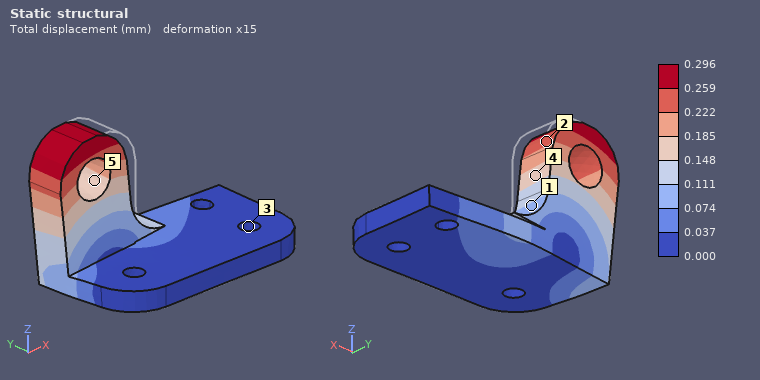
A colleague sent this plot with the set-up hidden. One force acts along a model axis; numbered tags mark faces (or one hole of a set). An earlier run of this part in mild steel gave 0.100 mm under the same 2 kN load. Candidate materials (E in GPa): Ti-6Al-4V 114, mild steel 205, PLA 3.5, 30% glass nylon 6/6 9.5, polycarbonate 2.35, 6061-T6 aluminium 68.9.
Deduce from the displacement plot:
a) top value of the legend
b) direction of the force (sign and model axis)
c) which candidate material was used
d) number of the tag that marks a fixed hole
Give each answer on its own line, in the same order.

0.296 mm
-X
6061-T6 aluminium
3
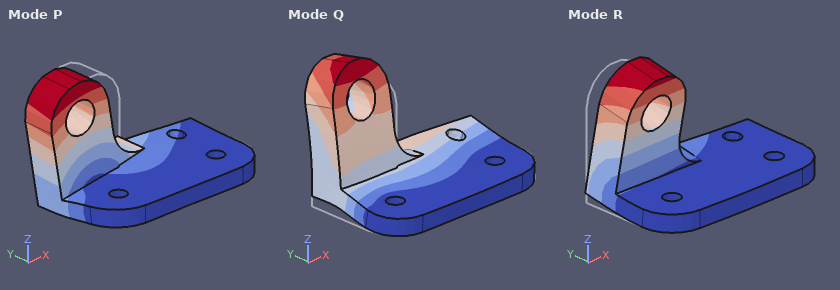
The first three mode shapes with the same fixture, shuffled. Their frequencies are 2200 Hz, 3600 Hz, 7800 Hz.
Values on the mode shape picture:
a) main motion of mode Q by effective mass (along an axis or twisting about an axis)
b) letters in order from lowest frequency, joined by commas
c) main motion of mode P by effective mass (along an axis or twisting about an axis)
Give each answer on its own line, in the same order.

along Z
R, P, Q
along X
